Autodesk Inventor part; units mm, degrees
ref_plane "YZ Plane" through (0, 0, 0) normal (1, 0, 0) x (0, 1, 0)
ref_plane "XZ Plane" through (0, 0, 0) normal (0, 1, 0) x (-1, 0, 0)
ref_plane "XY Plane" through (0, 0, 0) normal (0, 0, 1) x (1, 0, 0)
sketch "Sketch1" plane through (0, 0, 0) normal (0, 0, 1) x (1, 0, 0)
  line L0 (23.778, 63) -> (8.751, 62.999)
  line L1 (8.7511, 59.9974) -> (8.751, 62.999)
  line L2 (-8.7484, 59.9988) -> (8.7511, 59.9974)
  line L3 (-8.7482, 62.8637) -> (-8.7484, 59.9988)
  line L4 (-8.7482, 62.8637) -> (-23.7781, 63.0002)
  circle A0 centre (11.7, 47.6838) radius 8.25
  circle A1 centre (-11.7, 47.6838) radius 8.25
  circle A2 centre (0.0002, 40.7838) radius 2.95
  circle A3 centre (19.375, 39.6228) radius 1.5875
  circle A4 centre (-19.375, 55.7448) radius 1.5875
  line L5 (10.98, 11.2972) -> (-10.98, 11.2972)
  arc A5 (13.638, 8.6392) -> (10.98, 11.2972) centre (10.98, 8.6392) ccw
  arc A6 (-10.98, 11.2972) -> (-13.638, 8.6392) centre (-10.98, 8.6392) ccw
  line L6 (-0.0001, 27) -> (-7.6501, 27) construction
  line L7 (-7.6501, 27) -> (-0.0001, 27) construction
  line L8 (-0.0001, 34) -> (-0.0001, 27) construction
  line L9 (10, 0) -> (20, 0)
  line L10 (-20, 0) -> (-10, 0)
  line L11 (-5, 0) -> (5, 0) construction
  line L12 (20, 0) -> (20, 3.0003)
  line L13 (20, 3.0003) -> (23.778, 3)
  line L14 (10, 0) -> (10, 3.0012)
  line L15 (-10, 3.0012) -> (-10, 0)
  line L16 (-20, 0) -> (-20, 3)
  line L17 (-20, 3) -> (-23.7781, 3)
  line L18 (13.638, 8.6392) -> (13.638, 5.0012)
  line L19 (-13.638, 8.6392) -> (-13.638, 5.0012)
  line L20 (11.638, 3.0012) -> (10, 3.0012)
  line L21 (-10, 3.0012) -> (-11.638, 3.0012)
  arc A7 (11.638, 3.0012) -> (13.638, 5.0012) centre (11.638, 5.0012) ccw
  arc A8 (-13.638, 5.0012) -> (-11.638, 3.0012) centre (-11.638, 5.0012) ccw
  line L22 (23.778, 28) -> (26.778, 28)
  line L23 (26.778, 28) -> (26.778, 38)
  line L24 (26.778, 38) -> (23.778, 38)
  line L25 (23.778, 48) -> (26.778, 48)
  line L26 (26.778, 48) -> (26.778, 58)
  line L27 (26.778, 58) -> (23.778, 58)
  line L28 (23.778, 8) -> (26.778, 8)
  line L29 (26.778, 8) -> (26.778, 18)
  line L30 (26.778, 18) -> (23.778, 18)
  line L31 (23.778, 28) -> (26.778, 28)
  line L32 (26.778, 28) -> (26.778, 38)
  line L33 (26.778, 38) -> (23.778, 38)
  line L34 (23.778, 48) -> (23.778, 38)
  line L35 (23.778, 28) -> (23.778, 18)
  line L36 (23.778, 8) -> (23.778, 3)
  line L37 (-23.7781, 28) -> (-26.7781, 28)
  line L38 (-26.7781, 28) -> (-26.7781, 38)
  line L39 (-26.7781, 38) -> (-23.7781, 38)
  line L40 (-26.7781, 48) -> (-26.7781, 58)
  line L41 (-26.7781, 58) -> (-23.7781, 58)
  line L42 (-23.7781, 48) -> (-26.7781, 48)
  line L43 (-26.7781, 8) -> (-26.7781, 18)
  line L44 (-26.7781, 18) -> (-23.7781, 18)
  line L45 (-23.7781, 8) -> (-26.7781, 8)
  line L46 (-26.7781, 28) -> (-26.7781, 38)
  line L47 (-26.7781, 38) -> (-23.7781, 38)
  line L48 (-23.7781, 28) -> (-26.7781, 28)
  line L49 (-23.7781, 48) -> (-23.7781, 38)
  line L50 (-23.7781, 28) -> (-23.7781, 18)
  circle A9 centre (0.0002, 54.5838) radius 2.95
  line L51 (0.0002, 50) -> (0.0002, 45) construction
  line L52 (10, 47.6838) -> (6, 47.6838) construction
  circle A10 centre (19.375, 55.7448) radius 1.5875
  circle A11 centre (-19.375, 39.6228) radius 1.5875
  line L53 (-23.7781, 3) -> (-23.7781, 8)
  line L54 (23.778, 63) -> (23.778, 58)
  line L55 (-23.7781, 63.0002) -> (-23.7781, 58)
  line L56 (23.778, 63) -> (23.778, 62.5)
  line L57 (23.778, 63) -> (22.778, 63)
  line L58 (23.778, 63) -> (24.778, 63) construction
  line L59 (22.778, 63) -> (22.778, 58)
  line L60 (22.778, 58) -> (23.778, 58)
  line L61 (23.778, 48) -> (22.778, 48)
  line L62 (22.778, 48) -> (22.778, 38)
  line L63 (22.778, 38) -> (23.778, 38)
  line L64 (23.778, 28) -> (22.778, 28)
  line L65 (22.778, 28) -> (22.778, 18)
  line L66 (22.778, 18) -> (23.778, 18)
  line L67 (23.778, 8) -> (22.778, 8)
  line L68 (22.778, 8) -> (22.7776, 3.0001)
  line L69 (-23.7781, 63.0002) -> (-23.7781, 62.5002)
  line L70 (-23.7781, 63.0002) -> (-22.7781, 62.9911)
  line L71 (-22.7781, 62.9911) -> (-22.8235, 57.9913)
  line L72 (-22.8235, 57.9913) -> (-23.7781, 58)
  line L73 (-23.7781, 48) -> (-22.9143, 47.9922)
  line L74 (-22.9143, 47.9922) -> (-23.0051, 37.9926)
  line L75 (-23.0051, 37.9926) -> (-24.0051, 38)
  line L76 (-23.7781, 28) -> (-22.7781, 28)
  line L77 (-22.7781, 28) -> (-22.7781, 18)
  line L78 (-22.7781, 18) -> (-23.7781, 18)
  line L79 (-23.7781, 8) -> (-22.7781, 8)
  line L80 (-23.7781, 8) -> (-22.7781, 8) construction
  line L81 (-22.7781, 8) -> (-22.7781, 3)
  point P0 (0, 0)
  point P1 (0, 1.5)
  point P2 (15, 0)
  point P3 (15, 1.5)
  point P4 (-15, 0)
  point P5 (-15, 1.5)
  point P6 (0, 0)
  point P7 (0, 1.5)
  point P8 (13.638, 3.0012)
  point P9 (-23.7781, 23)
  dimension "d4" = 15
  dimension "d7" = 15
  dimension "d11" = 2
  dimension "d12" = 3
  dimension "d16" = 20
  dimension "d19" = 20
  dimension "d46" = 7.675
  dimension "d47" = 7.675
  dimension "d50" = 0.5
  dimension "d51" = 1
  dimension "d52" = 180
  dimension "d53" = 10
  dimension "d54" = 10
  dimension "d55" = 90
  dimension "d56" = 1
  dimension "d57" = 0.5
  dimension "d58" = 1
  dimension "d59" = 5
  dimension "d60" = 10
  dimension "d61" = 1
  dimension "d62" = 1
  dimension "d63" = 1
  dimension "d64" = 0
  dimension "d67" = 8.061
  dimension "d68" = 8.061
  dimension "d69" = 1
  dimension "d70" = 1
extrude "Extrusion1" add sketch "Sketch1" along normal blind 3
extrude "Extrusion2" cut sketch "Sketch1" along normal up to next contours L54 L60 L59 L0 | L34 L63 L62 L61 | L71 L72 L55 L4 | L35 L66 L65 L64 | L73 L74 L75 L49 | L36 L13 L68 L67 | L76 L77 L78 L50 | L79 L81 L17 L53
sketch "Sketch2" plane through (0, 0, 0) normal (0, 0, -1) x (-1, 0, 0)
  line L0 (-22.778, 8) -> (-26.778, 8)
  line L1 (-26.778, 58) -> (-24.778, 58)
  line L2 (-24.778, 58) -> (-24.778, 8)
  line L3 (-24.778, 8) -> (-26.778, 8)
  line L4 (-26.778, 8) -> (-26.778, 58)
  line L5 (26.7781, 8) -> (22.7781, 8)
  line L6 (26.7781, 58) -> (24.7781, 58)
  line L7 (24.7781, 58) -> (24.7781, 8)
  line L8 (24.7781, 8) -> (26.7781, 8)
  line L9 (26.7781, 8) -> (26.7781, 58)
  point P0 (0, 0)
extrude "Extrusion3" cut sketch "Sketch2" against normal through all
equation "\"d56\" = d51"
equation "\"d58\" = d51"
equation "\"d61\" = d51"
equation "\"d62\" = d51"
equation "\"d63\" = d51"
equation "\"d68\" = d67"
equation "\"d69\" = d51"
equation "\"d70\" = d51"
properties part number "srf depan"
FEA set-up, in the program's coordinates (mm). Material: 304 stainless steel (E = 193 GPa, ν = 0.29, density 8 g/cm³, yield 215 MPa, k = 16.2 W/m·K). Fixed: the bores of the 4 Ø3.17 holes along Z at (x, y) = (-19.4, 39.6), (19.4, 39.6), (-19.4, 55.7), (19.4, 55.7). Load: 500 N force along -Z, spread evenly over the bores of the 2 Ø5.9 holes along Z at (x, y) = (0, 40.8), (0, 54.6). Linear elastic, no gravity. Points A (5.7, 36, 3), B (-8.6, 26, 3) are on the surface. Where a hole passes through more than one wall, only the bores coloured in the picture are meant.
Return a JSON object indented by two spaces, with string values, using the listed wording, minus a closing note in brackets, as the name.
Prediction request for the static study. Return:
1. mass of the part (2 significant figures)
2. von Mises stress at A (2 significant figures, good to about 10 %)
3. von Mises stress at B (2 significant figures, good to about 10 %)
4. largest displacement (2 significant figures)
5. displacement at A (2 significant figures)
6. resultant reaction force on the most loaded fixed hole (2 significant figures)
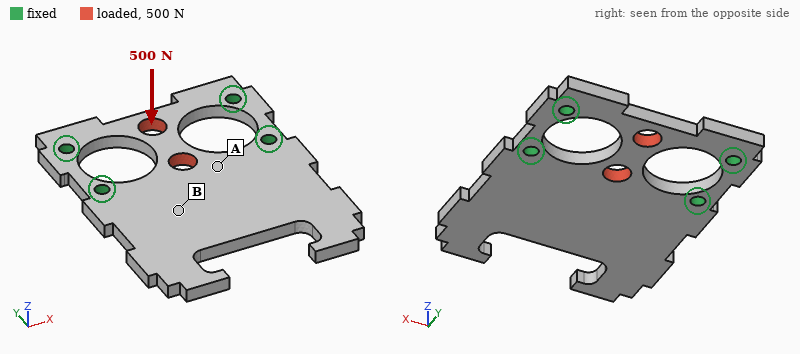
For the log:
{
  "mass of the part": "51 g",
  "von Mises stress at A": "45 MPa",
  "von Mises stress at B": "16 MPa",
  "largest displacement": "29 µm",
  "displacement at A": "12 µm",
  "resultant reaction force on the most loaded fixed hole": "130 N"
}
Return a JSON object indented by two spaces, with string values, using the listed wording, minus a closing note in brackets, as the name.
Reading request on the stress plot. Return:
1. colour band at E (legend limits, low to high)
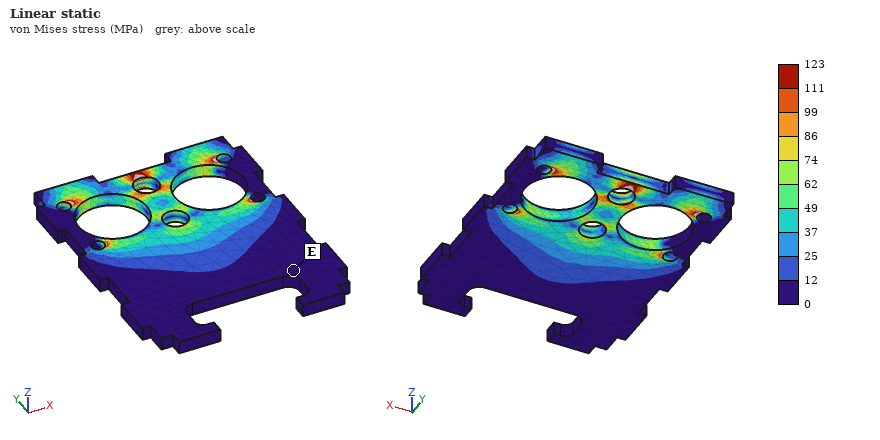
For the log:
{
  "colour band at E": "0 to 12 MPa"
}
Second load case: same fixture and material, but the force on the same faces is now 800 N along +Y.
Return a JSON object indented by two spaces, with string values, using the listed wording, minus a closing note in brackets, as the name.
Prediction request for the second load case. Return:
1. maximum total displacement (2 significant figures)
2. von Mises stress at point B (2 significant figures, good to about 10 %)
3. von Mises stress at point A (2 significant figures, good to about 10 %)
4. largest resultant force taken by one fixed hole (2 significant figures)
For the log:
{
  "maximum total displacement": "4.9 µm",
  "von Mises stress at point B": "8.0 MPa",
  "von Mises stress at point A": "13 MPa",
  "largest resultant force taken by one fixed hole": "330 N"
}
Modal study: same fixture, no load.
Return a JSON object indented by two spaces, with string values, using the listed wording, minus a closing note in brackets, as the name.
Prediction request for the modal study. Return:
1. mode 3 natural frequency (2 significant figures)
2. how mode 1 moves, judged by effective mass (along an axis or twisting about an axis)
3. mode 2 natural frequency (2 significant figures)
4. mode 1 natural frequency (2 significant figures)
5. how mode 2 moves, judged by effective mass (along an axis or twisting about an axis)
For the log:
{
  "mode 3 natural frequency": "6700 Hz",
  "how mode 1 moves, judged by effective mass": "along Z",
  "mode 2 natural frequency": "3000 Hz",
  "mode 1 natural frequency": "1600 Hz",
  "how mode 2 moves, judged by effective mass": "twisting about Y"
}
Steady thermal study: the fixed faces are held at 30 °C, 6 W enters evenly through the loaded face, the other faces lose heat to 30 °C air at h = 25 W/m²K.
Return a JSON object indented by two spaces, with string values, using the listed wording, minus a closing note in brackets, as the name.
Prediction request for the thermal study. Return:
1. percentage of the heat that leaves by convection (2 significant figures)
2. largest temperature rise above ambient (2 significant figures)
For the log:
{
  "percentage of the heat that leaves by convection": "35 %",
  "largest temperature rise above ambient": "72 K"
}
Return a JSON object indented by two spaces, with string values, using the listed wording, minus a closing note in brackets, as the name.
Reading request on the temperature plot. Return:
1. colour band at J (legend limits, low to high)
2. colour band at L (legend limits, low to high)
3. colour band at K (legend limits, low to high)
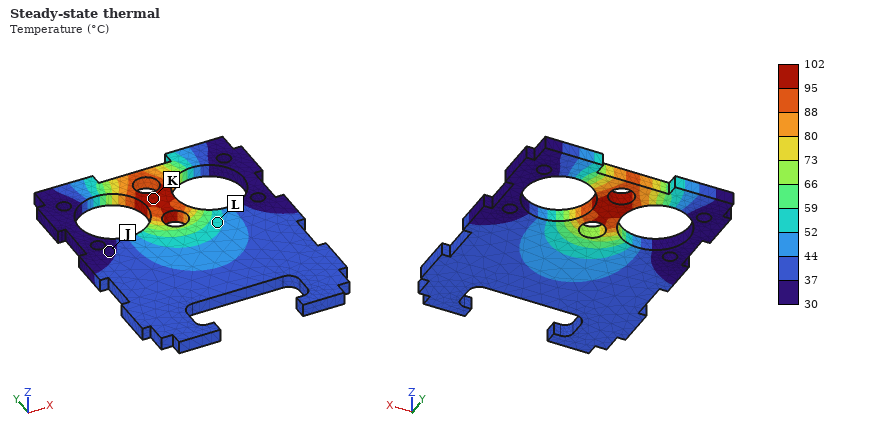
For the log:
{
  "colour band at J": "30 to 37 °C",
  "colour band at L": "52 to 59 °C",
  "colour band at K": "95 to 102 °C"
}
